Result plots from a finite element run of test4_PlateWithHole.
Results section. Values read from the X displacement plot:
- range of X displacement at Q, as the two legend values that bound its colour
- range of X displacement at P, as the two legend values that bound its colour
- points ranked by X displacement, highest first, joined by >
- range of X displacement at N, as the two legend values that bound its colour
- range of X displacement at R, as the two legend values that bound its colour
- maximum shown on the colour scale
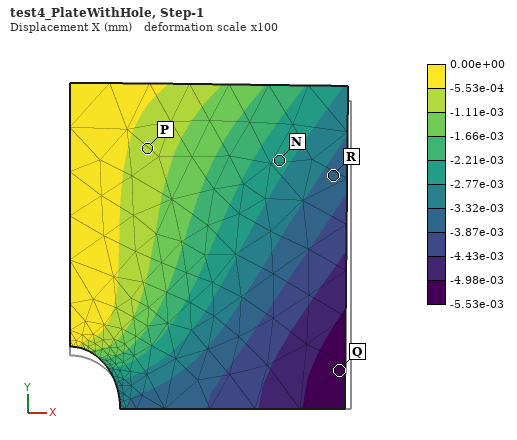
-5.53e-03 to -4.98e-03 mm
-1.11e-03 to -5.53e-04 mm
P > N > R > Q
-2.77e-03 to -2.21e-03 mm
-3.87e-03 to -3.32e-03 mm
0.00e+00 mm
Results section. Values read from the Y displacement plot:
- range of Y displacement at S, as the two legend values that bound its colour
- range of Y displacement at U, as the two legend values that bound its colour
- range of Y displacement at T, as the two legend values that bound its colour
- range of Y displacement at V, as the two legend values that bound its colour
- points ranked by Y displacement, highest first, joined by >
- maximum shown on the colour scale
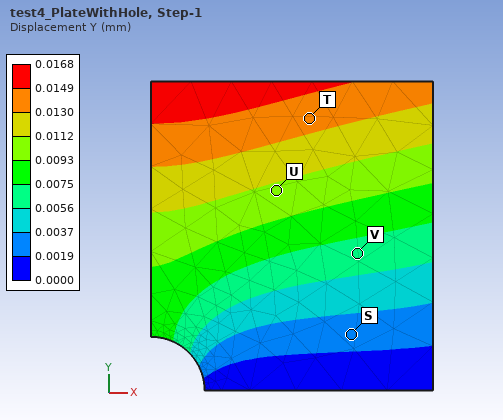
0.0019 to 0.0037 mm
0.0093 to 0.0112 mm
0.0130 to 0.0149 mm
0.0056 to 0.0075 mm
T > U > V > S
0.0168 mm
